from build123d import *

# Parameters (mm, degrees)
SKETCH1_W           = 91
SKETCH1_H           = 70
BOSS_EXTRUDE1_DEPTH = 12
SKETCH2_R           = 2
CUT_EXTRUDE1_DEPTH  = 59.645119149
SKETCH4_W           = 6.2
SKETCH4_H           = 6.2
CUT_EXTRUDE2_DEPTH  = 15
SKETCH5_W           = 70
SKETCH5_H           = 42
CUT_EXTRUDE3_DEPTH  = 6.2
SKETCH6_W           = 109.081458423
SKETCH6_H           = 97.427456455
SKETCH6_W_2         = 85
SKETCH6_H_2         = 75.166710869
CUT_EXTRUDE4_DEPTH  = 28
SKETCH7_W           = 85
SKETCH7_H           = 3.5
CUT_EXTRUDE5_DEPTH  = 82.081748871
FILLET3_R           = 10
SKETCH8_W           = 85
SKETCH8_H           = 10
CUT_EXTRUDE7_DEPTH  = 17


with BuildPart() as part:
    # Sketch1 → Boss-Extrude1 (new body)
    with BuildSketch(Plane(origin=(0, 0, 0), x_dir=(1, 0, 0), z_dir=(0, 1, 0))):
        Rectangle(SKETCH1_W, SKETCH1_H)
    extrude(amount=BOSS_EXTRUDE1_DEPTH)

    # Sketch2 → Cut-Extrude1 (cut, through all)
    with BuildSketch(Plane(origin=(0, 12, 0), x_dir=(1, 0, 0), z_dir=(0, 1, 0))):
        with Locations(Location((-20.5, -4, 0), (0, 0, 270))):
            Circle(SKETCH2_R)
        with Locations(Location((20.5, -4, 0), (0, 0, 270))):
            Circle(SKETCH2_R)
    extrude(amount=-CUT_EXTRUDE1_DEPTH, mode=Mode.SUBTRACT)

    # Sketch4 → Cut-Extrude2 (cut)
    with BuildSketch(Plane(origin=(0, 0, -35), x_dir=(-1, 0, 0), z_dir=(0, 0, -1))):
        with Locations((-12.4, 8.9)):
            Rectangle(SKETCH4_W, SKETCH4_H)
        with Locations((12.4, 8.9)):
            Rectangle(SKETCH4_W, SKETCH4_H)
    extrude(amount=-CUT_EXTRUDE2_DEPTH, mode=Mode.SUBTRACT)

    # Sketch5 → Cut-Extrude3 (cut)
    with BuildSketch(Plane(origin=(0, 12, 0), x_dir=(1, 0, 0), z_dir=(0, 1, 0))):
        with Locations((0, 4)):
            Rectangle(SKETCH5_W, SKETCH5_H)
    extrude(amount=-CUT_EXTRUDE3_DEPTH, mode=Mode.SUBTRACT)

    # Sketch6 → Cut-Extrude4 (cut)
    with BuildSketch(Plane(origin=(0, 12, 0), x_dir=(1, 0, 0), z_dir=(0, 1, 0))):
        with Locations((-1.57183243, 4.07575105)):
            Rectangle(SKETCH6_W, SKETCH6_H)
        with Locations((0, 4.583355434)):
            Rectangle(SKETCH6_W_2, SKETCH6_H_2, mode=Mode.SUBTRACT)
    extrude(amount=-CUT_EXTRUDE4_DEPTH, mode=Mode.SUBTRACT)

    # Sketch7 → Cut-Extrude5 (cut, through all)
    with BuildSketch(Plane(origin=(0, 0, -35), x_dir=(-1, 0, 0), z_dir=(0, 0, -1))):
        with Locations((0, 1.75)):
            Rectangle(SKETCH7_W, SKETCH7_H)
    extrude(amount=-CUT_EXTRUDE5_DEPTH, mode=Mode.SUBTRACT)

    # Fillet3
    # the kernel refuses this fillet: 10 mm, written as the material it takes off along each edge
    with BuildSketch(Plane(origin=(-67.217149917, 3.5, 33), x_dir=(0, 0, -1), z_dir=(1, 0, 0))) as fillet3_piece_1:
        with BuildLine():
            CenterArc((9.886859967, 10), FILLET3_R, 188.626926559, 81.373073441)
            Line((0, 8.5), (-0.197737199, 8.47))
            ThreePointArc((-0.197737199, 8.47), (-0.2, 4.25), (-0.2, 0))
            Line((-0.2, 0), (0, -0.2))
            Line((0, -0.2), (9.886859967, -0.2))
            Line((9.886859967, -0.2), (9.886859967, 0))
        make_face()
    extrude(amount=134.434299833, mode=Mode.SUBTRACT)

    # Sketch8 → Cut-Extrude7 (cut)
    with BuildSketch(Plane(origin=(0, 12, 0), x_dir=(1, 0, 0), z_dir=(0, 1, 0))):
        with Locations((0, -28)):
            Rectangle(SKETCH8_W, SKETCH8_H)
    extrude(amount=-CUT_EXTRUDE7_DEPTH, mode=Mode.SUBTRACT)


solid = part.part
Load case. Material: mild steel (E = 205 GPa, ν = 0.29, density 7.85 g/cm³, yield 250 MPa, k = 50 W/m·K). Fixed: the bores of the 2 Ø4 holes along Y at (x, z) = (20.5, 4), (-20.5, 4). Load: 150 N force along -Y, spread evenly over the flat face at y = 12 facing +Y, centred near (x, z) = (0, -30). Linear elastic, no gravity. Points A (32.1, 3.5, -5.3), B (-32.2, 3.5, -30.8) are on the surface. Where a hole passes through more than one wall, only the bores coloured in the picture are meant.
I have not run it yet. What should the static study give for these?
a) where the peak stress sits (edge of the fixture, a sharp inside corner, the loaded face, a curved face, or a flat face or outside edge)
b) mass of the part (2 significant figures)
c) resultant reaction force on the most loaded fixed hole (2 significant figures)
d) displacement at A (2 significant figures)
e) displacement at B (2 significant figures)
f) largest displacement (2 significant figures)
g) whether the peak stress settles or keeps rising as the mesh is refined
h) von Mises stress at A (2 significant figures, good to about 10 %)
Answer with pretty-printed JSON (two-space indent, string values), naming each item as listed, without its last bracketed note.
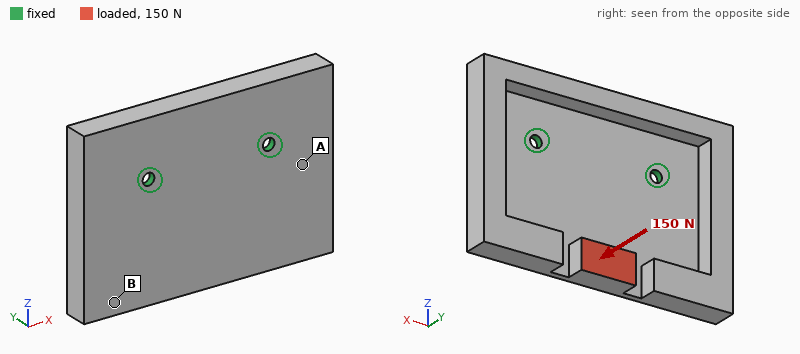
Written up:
{
  "where the peak stress sits": "edge of the fixture",
  "mass of the part": "180 g",
  "resultant reaction force on the most loaded fixed hole": "75 N",
  "displacement at A": "16 µm",
  "displacement at B": "64 µm",
  "largest displacement": "87 µm",
  "whether the peak stress settles or keeps rising as the mesh is refined": "keeps rising",
  "von Mises stress at A": "22 MPa"
}
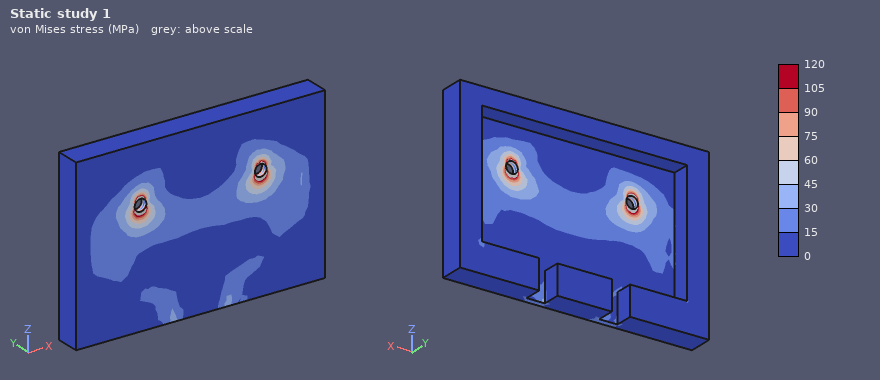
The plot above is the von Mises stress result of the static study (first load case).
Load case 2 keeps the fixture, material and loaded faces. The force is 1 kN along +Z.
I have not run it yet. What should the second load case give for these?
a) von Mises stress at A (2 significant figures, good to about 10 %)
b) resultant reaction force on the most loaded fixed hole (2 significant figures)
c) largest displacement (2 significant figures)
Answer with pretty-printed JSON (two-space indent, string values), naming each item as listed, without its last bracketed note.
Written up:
{
  "von Mises stress at A": "34 MPa",
  "resultant reaction force on the most loaded fixed hole": "520 N",
  "largest displacement": "0.16 mm"
}
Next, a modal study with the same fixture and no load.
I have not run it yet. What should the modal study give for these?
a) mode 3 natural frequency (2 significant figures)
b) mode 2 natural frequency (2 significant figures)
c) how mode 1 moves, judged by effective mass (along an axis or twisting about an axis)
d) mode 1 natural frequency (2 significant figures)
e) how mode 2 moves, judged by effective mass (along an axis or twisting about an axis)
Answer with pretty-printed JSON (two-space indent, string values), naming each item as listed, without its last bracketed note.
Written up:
{
  "mode 3 natural frequency": "2700 Hz",
  "mode 2 natural frequency": "1600 Hz",
  "how mode 1 moves, judged by effective mass": "along Y",
  "mode 1 natural frequency": "880 Hz",
  "how mode 2 moves, judged by effective mass": "twisting about Z"
}
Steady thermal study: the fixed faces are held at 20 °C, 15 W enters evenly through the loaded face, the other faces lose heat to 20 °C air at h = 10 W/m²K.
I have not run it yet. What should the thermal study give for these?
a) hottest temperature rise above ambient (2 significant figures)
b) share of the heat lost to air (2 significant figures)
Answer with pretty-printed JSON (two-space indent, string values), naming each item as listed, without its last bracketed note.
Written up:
{
  "hottest temperature rise above ambient": "80 K",
  "share of the heat lost to air": "22 %"
}
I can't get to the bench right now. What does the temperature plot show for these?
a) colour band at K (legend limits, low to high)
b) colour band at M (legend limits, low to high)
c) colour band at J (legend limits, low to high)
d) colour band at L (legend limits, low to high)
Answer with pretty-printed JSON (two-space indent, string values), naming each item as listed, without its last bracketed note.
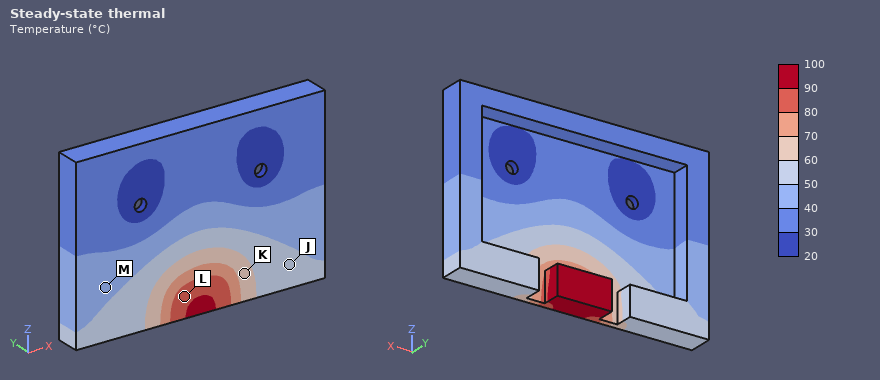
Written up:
{
  "colour band at K": "60 to 70 °C",
  "colour band at M": "40 to 50 °C",
  "colour band at J": "50 to 60 °C",
  "colour band at L": "80 to 90 °C"
}
